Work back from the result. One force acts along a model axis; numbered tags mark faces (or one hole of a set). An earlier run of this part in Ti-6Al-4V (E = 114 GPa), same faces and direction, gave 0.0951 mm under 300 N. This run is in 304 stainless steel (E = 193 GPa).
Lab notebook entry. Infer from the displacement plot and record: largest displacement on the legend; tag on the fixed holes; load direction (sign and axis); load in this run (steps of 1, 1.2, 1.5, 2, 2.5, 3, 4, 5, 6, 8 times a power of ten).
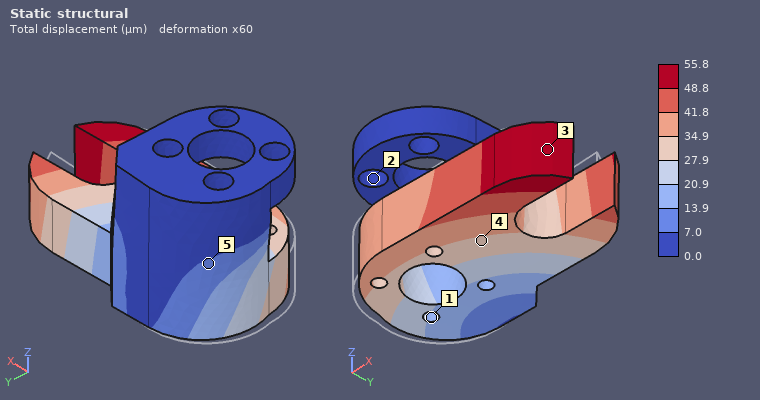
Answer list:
55.8 µm
2
+X
300 N
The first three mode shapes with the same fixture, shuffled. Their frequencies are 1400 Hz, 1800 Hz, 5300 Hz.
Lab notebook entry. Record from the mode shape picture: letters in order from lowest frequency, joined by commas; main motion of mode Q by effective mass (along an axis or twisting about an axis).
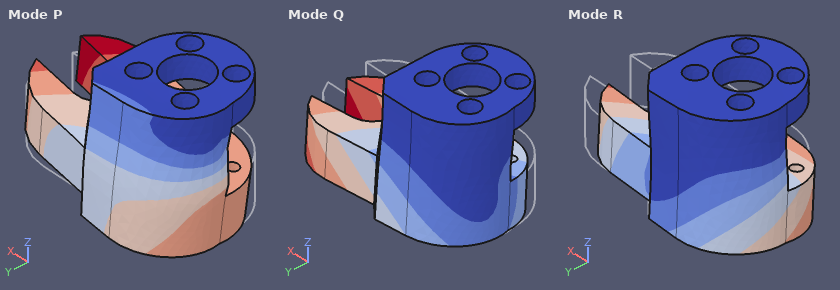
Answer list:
Q, R, P
along Y
